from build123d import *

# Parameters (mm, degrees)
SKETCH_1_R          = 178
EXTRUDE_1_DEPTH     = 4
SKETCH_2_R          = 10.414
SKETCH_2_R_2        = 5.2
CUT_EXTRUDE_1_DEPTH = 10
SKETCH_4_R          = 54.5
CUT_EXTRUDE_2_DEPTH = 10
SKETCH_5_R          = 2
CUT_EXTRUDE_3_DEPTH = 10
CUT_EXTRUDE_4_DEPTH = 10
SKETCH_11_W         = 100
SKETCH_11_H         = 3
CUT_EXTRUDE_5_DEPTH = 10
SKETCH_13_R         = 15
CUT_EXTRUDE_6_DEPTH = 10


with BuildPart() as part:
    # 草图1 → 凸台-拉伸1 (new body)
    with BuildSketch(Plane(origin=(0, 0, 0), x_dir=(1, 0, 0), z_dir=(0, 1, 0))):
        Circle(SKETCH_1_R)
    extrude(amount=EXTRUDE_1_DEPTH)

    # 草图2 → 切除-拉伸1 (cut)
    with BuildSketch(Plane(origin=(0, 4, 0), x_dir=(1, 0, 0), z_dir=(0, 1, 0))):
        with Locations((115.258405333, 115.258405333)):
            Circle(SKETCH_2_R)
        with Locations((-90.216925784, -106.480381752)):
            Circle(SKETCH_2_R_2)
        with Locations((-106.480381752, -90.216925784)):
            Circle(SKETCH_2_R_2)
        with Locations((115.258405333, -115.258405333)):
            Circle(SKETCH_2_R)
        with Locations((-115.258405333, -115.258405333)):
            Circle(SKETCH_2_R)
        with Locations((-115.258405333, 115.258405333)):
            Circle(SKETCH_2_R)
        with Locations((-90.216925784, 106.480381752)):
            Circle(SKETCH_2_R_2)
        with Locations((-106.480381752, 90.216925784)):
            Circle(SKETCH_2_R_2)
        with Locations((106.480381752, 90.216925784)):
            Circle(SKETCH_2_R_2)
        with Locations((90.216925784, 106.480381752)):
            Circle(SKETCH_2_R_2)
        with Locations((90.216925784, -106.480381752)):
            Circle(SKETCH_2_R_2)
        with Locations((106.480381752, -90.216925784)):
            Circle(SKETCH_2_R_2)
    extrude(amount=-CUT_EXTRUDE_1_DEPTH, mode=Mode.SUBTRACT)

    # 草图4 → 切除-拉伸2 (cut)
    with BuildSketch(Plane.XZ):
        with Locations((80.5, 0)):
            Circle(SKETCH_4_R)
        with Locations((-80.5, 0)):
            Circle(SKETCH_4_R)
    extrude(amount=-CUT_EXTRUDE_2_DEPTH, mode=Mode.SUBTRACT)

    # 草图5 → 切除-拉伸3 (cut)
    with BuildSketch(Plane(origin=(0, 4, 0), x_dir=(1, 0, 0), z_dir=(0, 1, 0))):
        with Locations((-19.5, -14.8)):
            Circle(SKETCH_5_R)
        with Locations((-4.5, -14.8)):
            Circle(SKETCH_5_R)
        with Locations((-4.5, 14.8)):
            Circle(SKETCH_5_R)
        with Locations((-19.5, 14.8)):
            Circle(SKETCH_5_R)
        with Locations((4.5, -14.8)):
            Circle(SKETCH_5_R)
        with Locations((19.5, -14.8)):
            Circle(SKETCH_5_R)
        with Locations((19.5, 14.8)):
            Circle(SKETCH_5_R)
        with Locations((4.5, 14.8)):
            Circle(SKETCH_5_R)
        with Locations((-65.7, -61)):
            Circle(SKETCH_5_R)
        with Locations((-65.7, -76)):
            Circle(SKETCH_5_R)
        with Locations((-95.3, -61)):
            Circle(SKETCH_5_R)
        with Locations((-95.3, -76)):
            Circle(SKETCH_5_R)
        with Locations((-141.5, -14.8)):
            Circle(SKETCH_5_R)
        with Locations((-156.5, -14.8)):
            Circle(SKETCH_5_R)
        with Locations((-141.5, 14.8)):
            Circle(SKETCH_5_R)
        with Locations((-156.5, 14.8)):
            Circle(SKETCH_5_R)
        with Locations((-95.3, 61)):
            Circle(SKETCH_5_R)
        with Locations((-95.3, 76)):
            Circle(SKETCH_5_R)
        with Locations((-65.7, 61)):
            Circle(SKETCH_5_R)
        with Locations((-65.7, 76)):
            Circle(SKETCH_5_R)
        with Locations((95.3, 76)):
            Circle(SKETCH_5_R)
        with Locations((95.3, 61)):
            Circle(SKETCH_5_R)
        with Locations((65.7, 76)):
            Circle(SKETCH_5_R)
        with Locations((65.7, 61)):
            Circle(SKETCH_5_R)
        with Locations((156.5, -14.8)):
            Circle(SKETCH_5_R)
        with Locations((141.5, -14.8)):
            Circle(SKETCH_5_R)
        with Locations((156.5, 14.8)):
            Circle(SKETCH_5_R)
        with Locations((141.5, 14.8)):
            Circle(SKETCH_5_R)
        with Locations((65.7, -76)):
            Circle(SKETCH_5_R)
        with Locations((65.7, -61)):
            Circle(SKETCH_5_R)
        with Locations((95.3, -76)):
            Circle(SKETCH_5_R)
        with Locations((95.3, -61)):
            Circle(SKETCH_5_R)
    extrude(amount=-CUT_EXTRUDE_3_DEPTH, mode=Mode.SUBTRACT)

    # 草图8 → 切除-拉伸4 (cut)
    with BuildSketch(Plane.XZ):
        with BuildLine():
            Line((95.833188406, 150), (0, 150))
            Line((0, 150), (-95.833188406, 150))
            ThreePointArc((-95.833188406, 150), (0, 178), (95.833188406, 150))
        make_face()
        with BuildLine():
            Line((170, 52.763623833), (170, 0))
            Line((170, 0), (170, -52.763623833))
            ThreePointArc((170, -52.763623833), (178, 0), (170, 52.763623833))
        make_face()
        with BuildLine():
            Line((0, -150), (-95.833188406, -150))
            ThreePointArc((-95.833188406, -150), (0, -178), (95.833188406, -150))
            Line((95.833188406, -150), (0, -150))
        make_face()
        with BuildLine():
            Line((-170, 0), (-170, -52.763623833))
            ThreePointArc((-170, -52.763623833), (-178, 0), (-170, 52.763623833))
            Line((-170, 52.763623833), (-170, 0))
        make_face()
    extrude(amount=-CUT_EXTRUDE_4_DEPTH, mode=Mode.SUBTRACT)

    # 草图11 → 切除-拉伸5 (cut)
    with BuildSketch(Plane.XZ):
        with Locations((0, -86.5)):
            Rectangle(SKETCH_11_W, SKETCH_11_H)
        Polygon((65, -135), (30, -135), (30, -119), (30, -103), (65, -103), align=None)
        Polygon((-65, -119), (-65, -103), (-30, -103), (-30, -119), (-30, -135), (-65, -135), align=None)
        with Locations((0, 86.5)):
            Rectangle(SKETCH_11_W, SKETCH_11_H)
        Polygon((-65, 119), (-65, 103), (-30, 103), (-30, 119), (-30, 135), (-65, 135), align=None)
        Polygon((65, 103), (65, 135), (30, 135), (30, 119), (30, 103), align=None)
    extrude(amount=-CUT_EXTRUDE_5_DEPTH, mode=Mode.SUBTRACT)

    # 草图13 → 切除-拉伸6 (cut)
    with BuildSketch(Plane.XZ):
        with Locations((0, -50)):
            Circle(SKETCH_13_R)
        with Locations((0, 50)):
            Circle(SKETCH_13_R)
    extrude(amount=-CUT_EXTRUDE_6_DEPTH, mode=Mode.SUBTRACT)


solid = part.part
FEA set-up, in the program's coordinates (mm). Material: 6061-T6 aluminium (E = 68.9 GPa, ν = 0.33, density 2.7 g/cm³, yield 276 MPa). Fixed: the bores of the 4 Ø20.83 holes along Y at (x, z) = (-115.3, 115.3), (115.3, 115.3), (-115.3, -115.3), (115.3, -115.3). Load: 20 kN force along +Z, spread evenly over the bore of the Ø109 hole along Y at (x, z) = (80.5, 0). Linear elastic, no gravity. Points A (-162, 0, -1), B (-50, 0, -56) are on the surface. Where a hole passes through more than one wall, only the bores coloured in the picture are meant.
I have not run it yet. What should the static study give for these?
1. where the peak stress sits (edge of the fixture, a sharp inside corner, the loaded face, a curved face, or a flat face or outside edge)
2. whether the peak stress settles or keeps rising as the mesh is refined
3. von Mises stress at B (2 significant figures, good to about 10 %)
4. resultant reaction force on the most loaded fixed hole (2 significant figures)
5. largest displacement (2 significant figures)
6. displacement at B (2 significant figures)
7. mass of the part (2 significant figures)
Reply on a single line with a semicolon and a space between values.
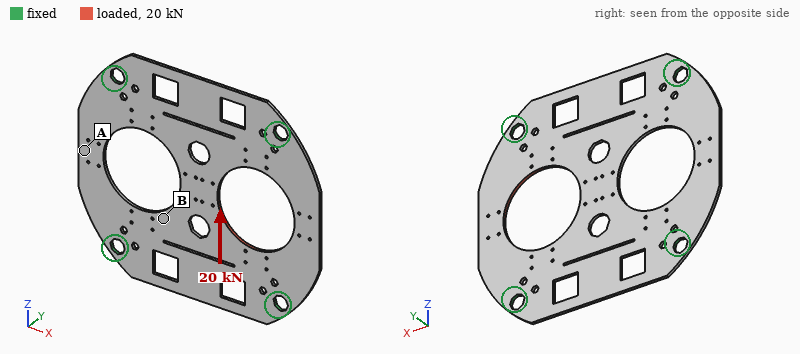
a sharp inside corner; keeps rising; 19 MPa; 8.1 kN; 75 µm; 29 µm; 690 g
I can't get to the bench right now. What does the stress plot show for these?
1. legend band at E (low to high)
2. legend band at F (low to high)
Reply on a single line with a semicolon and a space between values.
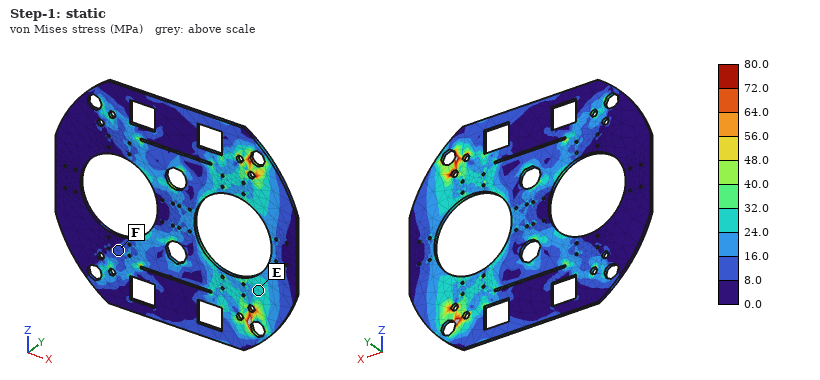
24.0 to 32.0 MPa; 8.0 to 16.0 MPa
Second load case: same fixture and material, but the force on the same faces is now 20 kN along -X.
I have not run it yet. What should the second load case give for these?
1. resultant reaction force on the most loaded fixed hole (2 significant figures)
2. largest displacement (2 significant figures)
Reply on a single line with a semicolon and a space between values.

6.5 kN; 0.12 mm
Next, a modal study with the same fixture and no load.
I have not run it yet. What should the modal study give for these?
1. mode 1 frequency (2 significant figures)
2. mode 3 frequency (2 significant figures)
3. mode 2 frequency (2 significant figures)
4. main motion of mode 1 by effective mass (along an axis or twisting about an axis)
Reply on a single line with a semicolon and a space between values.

300 Hz; 420 Hz; 410 Hz; along Y
